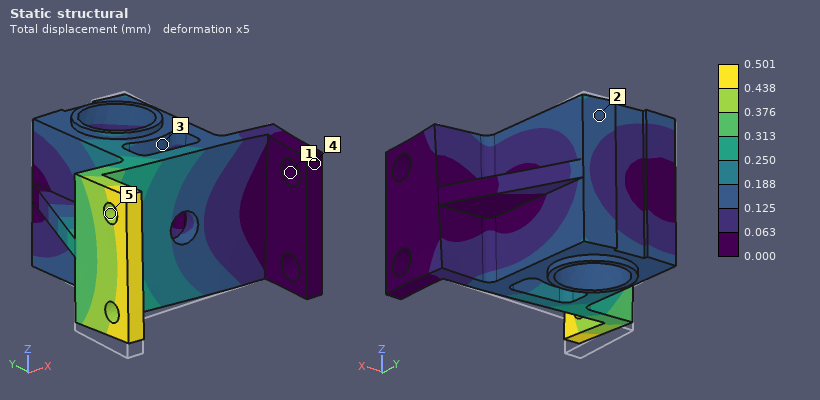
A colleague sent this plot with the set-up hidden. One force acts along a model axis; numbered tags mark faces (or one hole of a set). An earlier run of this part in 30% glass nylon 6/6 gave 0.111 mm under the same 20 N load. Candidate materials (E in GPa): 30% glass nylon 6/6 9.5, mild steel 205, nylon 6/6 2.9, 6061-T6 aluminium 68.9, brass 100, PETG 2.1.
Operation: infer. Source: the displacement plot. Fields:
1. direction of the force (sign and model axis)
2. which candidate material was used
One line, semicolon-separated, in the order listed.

+Z; PETG
